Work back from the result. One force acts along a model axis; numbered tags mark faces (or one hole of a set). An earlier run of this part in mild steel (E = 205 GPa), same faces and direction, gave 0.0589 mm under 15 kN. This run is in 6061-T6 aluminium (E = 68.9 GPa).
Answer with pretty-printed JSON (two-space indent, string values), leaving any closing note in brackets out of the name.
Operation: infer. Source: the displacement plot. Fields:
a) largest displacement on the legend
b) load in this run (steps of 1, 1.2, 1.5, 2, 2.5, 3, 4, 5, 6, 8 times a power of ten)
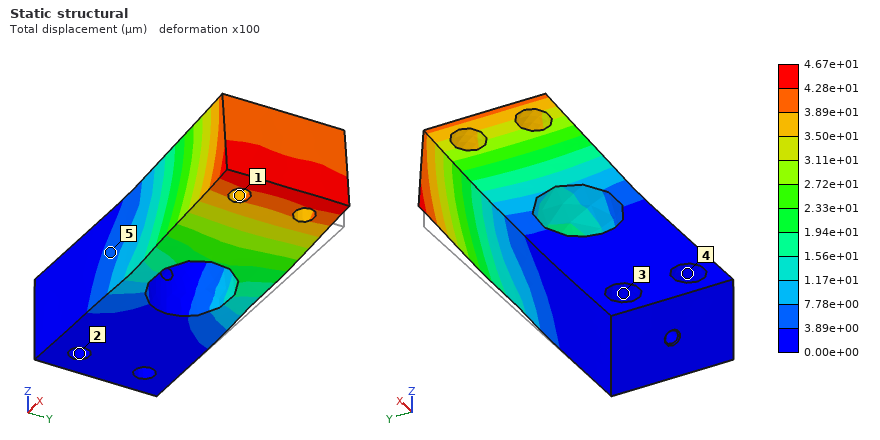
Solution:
{
  "largest displacement on the legend": "4.67e+01 µm",
  "load in this run": "4 kN"
}
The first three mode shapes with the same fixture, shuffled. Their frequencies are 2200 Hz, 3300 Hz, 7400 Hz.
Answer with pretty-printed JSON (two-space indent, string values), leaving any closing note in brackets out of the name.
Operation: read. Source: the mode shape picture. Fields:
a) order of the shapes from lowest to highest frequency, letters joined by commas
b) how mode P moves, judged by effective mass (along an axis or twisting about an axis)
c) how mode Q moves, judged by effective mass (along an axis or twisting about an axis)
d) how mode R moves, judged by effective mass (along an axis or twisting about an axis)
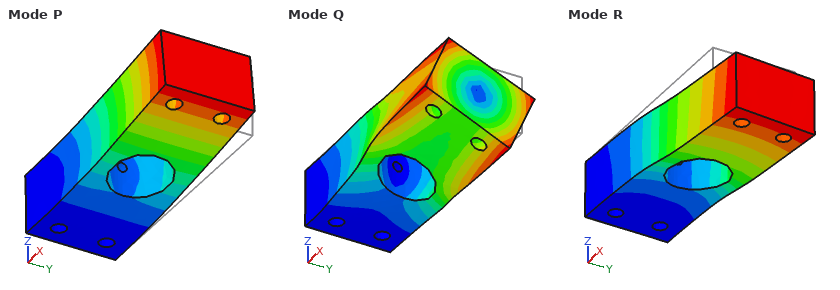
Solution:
{
  "order of the shapes from lowest to highest frequency, letters joined by commas": "P, R, Q",
  "how mode P moves, judged by effective mass": "along Z",
  "how mode Q moves, judged by effective mass": "twisting about X",
  "how mode R moves, judged by effective mass": "along Y"
}
